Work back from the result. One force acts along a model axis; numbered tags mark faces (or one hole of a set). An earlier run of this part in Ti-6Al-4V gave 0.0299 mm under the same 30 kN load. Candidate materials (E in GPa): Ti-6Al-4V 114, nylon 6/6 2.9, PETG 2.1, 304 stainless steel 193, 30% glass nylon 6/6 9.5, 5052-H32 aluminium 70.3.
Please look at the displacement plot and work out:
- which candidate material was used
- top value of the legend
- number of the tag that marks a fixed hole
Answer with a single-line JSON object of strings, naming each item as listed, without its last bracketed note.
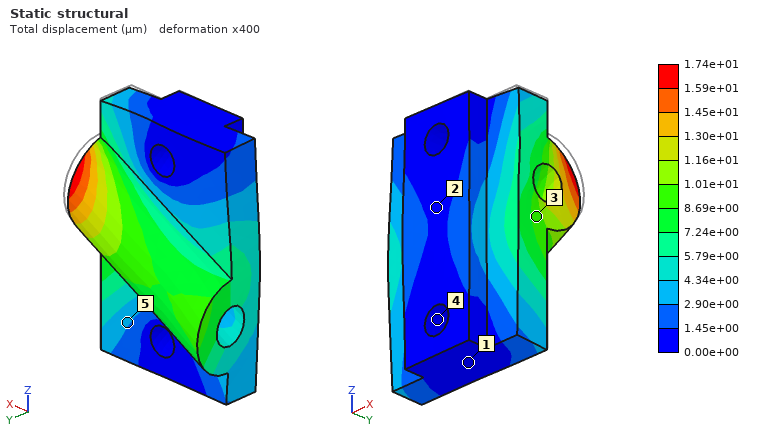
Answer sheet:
{"which candidate material was used": "304 stainless steel", "top value of the legend": "1.74e+01 µm", "number of the tag that marks a fixed hole": "4"}
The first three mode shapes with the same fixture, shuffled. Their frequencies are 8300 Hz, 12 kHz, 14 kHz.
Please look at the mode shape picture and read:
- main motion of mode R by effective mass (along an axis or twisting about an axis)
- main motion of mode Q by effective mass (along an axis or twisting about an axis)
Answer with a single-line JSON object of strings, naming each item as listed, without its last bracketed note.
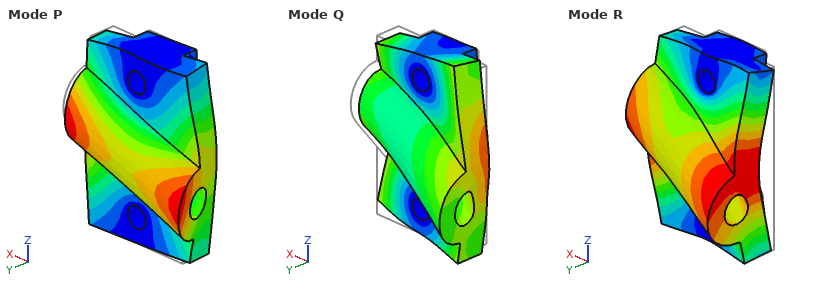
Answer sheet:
{"main motion of mode R by effective mass": "along Y", "main motion of mode Q by effective mass": "along X"}
